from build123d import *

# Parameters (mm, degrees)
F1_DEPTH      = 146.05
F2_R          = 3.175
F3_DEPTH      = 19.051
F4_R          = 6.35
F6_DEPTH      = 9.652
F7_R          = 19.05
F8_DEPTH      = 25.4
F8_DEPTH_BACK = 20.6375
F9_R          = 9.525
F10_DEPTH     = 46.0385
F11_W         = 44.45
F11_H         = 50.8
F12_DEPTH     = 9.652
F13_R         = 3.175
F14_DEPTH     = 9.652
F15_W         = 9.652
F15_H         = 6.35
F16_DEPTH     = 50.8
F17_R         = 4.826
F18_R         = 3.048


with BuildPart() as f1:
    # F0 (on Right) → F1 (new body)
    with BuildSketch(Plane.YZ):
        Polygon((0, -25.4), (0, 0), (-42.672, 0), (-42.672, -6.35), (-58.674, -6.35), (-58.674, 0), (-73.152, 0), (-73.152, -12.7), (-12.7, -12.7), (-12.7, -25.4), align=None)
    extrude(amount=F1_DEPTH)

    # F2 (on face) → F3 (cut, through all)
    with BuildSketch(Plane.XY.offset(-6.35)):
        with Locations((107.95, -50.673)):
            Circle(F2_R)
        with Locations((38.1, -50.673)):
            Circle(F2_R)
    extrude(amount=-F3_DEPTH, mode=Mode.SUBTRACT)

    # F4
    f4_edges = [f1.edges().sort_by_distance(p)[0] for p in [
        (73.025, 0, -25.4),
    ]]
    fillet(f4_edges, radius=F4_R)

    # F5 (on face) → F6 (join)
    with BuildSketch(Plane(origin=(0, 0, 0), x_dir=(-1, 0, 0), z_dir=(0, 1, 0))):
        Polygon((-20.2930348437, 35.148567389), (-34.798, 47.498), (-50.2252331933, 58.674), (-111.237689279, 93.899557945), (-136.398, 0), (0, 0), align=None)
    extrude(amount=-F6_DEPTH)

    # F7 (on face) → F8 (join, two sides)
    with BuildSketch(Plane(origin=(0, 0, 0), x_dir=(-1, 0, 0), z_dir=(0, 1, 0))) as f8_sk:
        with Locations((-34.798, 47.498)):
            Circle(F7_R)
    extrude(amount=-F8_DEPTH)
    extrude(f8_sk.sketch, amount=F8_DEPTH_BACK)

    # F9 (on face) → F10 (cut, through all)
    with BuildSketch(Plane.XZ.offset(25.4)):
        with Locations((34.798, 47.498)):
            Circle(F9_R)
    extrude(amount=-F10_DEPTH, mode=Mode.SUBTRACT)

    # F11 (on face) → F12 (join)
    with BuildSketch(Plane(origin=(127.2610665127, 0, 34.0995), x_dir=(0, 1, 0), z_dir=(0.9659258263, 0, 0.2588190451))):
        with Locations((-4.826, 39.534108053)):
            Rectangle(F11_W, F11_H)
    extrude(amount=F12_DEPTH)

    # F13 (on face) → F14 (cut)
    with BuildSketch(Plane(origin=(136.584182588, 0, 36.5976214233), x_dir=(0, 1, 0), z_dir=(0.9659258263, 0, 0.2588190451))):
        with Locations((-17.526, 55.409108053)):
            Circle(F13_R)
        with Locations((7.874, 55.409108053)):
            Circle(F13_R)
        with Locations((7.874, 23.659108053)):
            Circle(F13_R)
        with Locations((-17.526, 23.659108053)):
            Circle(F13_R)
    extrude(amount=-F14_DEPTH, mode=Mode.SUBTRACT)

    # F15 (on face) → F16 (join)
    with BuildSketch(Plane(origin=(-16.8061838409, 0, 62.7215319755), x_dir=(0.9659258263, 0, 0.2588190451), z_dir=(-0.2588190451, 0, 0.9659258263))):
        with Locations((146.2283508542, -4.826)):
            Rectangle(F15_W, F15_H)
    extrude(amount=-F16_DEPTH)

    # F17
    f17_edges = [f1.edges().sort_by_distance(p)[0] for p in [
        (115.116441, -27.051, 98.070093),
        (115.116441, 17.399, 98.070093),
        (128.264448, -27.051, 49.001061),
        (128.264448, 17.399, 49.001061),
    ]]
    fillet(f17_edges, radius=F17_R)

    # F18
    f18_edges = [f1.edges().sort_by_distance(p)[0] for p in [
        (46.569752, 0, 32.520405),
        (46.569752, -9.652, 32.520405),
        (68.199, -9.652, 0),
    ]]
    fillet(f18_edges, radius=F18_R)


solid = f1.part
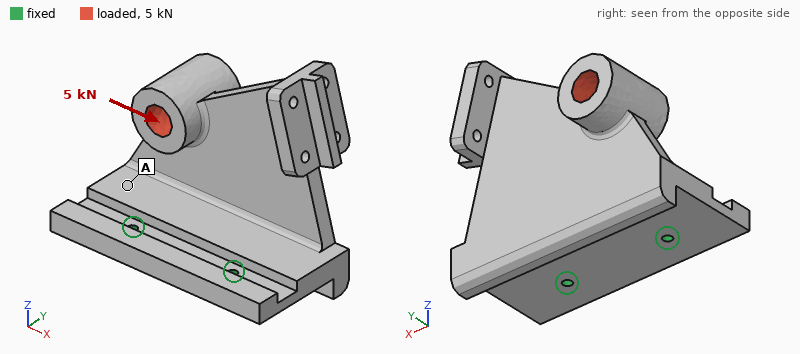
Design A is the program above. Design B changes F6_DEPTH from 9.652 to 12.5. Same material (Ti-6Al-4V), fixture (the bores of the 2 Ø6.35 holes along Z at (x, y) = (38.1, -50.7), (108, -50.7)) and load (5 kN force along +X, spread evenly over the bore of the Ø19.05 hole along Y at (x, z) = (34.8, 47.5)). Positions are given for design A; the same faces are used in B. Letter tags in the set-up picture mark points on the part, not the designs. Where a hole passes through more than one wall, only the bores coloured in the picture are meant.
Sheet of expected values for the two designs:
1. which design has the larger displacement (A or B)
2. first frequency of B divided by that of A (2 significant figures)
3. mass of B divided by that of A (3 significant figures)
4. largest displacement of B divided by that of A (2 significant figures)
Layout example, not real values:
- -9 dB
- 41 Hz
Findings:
- A
- 0.99
- 1.07
- 0.83
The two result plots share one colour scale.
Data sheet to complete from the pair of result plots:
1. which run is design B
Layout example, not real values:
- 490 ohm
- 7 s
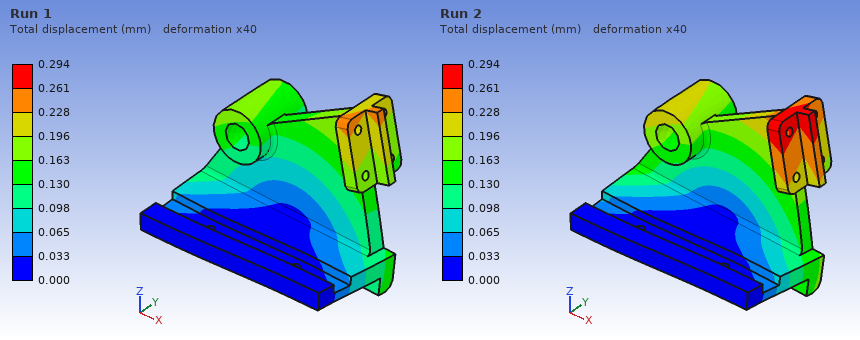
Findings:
- Run 1
